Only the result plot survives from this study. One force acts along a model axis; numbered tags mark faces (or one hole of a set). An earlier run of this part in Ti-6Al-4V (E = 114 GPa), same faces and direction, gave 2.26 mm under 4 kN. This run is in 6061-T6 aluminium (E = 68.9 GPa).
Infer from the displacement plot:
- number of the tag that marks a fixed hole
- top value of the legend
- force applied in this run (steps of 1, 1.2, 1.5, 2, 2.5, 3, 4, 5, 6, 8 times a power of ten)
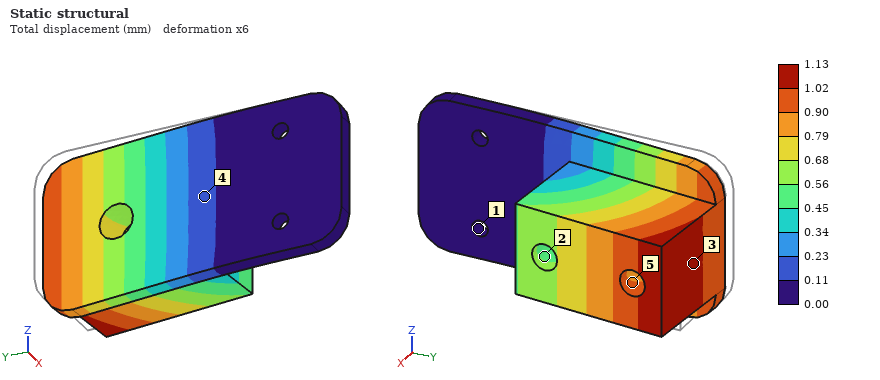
1
1.13 mm
1.2 kN
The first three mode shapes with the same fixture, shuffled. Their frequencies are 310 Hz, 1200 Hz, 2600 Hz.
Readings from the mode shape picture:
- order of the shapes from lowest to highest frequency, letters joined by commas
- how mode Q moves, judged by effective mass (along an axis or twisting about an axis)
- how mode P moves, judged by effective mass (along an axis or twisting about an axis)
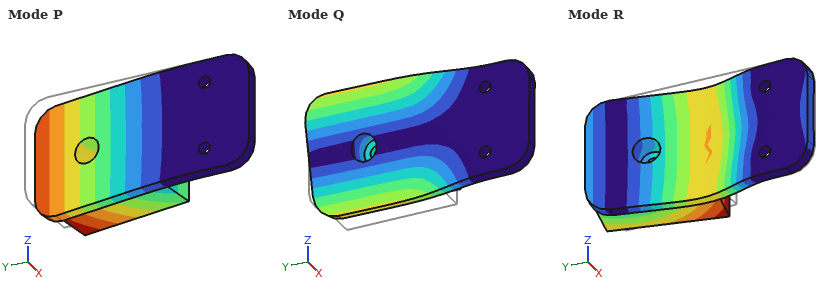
P, Q, R
along Z
along X
